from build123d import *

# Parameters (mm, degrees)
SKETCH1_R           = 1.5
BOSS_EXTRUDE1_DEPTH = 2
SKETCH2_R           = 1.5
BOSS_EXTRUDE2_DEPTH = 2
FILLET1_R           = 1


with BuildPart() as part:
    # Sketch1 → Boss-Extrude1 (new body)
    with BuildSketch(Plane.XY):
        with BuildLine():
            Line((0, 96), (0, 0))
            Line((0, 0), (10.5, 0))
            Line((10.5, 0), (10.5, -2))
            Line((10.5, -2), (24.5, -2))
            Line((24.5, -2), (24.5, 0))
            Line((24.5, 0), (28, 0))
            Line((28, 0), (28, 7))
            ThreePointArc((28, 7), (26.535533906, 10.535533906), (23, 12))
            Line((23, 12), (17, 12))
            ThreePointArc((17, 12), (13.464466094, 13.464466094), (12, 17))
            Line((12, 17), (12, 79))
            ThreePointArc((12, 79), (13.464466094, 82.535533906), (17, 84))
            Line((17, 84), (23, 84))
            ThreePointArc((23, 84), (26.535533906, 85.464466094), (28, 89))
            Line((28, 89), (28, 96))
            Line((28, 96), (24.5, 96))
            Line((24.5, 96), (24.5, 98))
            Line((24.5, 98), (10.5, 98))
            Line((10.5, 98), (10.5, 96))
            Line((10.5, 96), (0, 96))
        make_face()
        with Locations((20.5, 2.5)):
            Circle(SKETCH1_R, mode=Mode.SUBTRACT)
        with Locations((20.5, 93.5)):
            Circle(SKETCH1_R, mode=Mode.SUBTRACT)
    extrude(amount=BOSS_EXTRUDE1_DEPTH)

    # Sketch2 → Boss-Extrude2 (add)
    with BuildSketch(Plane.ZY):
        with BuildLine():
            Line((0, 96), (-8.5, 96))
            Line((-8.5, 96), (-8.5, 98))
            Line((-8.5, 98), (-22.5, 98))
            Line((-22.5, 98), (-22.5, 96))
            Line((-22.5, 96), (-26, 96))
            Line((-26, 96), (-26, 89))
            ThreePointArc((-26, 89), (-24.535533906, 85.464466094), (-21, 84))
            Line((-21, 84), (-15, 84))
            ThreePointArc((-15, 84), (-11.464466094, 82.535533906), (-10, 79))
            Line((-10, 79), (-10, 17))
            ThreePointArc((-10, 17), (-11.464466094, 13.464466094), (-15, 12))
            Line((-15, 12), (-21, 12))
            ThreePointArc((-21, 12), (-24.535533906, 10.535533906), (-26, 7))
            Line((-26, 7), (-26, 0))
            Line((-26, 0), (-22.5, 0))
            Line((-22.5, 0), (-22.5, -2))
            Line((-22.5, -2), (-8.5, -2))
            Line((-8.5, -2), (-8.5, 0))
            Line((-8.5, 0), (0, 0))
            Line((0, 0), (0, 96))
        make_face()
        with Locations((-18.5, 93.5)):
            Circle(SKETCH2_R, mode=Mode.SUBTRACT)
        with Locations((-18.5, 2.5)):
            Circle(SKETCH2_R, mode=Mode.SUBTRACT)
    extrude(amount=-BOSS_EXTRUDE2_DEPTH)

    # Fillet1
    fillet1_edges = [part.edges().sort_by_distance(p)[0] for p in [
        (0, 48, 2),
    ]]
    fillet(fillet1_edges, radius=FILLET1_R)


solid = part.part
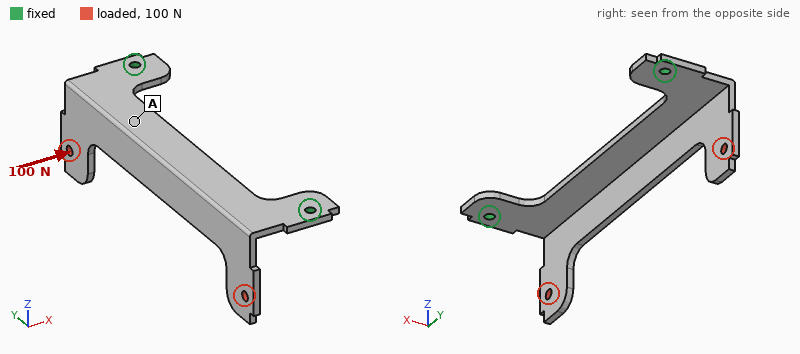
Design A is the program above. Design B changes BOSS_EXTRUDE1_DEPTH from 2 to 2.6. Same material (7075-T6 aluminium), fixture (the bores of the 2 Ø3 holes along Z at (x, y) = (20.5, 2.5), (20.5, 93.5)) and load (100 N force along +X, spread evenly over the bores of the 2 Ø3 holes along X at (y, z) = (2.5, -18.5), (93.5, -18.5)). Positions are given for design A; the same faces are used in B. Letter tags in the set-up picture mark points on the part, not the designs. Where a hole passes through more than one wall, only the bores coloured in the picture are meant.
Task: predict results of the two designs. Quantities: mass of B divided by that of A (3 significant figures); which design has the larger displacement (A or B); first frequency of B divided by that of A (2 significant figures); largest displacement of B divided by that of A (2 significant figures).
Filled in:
1.16
A
1.4
0.62
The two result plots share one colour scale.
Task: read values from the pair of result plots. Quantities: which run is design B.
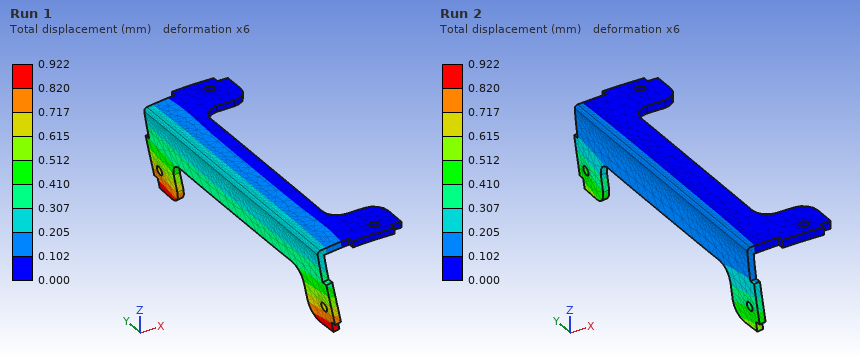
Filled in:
Run 2
